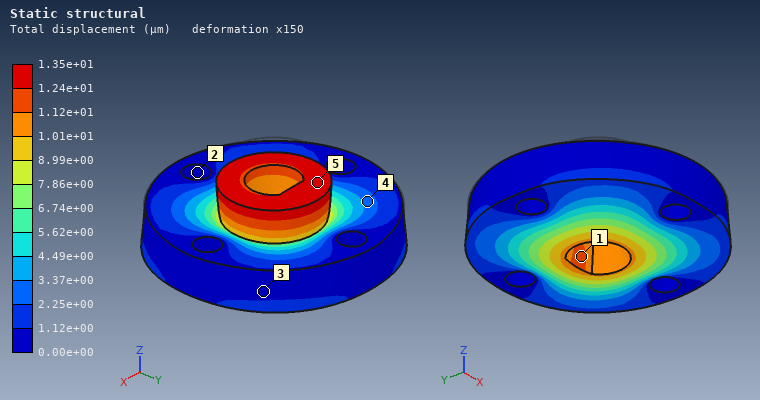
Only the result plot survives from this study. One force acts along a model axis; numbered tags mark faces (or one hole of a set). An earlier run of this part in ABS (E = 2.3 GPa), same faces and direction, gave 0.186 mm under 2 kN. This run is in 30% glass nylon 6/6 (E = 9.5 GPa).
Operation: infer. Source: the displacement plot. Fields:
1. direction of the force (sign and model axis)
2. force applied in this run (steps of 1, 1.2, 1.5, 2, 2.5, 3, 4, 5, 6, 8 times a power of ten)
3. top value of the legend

-Z
600 N
1.35e+01 µm
